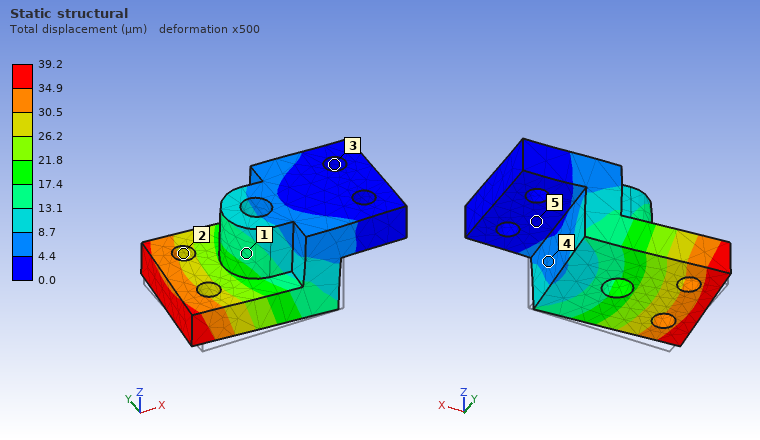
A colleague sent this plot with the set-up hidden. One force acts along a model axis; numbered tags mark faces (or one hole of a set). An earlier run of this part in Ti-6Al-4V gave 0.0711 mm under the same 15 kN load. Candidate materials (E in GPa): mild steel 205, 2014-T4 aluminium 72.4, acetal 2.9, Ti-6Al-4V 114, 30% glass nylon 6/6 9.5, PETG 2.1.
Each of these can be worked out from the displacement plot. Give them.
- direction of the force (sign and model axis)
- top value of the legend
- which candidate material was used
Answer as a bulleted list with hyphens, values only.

- +Y
- 39.2 µm
- mild steel
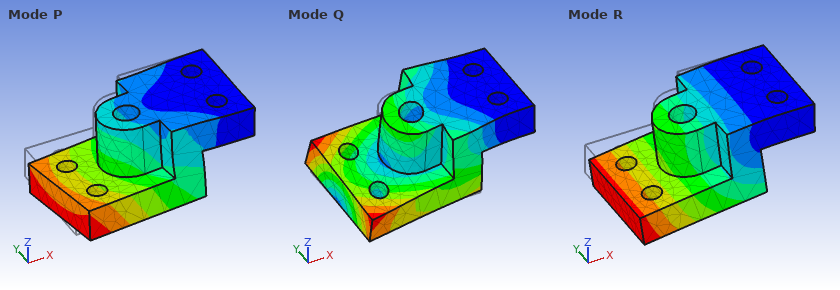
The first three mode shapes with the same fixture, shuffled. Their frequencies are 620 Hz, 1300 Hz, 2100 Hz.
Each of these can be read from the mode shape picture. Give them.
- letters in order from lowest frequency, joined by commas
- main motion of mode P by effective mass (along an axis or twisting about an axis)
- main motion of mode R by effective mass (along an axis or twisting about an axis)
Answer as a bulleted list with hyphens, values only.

- R, P, Q
- along Y
- along Z
